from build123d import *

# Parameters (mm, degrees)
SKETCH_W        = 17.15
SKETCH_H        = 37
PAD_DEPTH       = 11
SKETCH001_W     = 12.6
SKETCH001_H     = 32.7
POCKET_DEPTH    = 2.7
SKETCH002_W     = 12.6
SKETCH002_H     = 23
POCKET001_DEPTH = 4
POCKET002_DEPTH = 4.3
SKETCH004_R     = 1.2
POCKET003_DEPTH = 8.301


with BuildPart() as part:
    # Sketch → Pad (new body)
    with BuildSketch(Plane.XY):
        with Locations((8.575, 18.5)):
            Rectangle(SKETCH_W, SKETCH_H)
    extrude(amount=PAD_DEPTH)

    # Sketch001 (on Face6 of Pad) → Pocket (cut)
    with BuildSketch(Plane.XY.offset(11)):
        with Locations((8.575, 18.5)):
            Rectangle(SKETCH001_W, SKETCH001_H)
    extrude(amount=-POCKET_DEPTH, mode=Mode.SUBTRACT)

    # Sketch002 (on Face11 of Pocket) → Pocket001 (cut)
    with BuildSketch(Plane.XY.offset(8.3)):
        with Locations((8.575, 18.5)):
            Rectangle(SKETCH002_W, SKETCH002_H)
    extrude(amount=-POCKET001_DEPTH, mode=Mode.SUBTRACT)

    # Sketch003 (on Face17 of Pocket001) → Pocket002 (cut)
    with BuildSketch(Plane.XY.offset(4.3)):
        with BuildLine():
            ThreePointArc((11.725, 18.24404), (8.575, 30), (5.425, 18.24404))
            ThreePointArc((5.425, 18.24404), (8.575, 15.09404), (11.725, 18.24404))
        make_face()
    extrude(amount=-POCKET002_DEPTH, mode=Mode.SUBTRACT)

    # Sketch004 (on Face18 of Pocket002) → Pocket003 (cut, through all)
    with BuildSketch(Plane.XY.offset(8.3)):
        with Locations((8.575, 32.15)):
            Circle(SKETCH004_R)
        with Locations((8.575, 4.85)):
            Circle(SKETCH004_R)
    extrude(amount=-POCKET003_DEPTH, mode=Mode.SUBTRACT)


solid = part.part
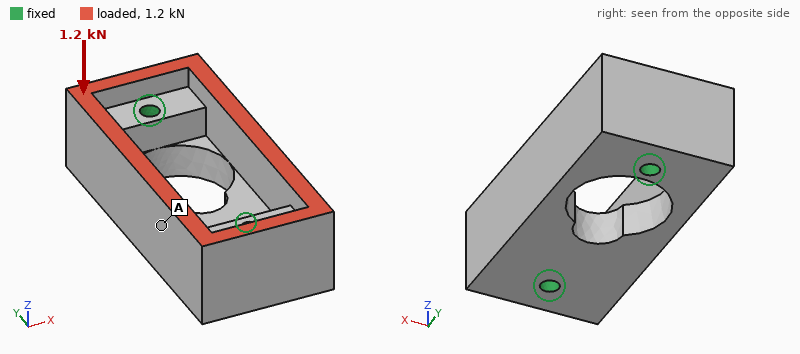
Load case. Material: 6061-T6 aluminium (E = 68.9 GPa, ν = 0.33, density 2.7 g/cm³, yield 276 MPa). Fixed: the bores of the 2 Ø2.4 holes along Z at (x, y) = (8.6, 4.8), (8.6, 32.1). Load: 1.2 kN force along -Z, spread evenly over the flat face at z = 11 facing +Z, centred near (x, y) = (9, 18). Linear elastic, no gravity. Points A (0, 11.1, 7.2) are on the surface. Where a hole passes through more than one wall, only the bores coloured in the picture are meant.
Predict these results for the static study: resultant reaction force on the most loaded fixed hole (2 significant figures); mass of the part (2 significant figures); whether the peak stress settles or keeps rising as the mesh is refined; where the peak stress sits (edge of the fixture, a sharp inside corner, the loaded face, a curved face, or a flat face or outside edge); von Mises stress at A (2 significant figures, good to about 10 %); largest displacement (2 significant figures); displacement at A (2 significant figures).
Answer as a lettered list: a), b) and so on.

a) 620 N
b) 11 g
c) keeps rising
d) edge of the fixture
e) 8.5 MPa
f) 6.5 µm
g) 4.4 µm
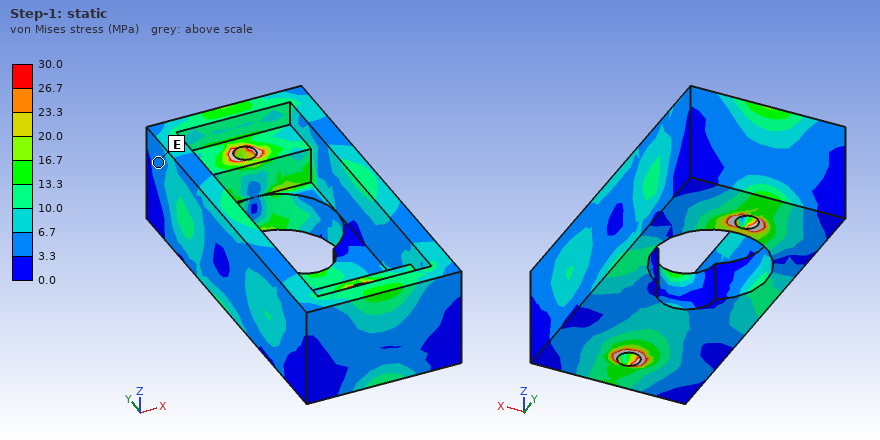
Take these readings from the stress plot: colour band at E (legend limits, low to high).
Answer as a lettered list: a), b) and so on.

a) 3.3 to 6.7 MPa
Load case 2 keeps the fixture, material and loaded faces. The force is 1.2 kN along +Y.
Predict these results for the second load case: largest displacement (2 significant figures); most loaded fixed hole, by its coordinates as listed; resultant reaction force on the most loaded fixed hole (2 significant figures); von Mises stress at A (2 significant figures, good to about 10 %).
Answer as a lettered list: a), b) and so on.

a) 5.6 µm
b) (8.6, 4.8)
c) 750 N
d) 9.1 MPa
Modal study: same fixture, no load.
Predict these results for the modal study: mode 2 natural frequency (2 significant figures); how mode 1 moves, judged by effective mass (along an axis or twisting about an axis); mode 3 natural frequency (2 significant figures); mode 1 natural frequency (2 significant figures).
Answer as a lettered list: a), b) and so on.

a) 26 kHz
b) along X
c) 27 kHz
d) 22 kHz
